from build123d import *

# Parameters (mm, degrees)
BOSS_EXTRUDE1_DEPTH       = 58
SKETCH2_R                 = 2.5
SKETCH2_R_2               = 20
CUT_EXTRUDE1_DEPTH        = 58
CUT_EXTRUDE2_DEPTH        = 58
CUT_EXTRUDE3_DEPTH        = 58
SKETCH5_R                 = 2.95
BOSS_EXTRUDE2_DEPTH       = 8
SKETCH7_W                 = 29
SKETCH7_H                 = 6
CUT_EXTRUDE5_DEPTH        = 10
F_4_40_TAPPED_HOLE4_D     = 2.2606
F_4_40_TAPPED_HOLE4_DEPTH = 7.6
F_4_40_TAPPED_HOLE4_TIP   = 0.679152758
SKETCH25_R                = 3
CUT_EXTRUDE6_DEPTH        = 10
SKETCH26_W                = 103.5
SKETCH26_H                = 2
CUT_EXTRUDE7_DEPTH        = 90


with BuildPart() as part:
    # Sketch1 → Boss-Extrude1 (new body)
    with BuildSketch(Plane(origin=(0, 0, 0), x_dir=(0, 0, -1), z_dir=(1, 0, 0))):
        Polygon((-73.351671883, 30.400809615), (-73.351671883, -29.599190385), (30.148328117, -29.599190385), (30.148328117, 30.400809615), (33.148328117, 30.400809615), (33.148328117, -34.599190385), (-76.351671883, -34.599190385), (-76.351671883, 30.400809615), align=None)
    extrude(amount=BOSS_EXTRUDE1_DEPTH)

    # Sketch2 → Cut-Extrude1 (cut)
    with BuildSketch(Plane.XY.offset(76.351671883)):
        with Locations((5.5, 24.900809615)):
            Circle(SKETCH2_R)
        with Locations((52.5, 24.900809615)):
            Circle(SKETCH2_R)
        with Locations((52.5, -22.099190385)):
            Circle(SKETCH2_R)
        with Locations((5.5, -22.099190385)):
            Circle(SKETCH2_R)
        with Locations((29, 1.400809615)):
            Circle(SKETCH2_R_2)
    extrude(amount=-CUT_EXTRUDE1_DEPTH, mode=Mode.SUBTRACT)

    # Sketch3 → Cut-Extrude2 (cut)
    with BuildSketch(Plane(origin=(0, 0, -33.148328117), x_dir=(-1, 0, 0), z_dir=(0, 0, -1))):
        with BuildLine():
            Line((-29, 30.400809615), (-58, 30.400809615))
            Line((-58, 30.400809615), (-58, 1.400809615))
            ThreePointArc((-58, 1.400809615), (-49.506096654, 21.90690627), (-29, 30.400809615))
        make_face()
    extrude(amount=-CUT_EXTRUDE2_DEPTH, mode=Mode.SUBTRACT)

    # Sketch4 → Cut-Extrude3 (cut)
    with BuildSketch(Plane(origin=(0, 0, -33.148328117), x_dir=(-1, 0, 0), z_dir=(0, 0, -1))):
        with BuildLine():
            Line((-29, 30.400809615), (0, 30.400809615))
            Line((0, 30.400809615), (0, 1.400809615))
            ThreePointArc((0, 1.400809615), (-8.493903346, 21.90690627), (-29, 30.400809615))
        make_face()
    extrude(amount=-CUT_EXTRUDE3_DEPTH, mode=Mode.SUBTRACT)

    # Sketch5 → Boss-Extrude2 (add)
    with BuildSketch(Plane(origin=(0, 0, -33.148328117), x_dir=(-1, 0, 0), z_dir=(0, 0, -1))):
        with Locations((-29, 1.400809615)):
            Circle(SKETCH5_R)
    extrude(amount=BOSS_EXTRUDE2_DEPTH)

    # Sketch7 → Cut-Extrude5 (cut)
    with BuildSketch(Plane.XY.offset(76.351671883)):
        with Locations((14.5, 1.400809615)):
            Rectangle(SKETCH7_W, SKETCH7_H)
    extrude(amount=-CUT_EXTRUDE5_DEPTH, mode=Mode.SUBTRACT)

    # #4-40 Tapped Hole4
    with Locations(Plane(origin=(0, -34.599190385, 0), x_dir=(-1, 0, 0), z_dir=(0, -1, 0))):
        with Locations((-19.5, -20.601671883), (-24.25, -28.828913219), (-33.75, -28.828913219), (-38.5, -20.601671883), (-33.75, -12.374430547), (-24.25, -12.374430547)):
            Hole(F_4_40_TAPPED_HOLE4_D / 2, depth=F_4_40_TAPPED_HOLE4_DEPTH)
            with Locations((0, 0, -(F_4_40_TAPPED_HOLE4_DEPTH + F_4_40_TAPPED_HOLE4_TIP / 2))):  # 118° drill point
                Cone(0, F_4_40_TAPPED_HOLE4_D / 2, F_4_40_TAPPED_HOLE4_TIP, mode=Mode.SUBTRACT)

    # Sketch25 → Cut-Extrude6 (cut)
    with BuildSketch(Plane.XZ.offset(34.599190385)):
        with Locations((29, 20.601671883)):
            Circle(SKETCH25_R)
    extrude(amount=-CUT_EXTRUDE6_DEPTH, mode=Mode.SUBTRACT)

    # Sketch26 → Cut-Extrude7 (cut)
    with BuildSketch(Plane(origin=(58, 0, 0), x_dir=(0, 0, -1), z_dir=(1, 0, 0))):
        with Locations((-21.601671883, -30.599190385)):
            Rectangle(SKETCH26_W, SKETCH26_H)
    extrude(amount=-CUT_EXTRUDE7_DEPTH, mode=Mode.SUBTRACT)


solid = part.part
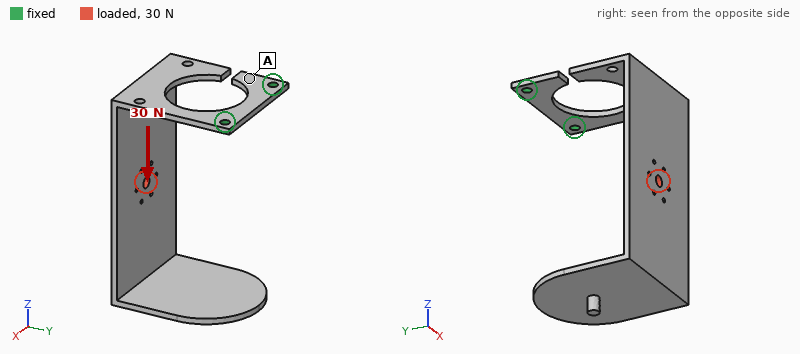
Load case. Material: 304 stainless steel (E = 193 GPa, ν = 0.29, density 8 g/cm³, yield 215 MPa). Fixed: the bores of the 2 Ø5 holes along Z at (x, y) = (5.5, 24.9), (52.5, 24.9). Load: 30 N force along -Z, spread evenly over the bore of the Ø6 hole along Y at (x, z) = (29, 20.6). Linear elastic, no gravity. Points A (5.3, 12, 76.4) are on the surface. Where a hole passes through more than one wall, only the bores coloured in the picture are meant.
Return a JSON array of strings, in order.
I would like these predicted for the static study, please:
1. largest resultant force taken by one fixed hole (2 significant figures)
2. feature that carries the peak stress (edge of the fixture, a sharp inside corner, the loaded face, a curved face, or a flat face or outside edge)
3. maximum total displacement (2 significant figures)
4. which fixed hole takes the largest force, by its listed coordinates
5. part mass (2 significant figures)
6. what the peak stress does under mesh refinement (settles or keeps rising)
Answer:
["31 N", "edge of the fixture", "1.3 mm", "(52.5, 24.9)", "280 g", "keeps rising"]
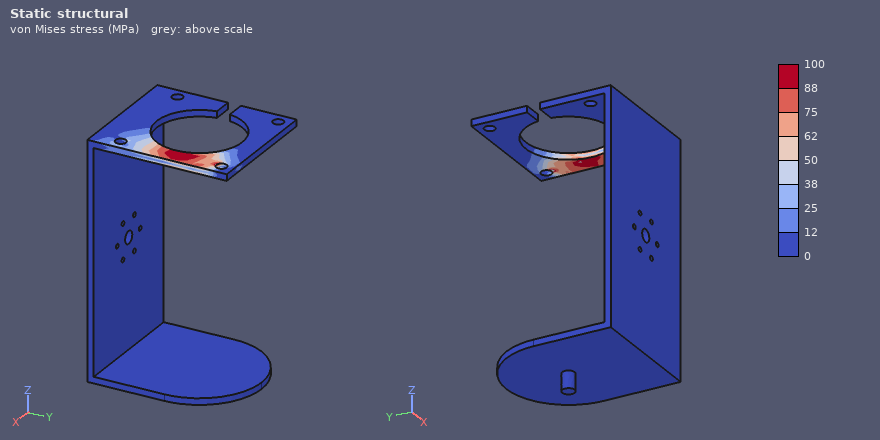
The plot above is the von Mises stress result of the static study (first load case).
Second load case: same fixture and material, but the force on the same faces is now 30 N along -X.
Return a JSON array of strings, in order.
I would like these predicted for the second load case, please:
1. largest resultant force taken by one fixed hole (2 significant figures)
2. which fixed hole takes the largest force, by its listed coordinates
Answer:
["33 N", "(52.5, 24.9)"]
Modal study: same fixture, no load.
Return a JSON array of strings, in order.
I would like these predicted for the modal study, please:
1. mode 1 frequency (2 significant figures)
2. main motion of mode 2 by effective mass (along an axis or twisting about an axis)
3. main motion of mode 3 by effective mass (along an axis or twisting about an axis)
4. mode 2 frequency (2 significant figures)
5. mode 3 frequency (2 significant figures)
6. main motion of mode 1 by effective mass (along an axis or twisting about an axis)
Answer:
["37 Hz", "along X", "along Z", "46 Hz", "170 Hz", "along Y"]
